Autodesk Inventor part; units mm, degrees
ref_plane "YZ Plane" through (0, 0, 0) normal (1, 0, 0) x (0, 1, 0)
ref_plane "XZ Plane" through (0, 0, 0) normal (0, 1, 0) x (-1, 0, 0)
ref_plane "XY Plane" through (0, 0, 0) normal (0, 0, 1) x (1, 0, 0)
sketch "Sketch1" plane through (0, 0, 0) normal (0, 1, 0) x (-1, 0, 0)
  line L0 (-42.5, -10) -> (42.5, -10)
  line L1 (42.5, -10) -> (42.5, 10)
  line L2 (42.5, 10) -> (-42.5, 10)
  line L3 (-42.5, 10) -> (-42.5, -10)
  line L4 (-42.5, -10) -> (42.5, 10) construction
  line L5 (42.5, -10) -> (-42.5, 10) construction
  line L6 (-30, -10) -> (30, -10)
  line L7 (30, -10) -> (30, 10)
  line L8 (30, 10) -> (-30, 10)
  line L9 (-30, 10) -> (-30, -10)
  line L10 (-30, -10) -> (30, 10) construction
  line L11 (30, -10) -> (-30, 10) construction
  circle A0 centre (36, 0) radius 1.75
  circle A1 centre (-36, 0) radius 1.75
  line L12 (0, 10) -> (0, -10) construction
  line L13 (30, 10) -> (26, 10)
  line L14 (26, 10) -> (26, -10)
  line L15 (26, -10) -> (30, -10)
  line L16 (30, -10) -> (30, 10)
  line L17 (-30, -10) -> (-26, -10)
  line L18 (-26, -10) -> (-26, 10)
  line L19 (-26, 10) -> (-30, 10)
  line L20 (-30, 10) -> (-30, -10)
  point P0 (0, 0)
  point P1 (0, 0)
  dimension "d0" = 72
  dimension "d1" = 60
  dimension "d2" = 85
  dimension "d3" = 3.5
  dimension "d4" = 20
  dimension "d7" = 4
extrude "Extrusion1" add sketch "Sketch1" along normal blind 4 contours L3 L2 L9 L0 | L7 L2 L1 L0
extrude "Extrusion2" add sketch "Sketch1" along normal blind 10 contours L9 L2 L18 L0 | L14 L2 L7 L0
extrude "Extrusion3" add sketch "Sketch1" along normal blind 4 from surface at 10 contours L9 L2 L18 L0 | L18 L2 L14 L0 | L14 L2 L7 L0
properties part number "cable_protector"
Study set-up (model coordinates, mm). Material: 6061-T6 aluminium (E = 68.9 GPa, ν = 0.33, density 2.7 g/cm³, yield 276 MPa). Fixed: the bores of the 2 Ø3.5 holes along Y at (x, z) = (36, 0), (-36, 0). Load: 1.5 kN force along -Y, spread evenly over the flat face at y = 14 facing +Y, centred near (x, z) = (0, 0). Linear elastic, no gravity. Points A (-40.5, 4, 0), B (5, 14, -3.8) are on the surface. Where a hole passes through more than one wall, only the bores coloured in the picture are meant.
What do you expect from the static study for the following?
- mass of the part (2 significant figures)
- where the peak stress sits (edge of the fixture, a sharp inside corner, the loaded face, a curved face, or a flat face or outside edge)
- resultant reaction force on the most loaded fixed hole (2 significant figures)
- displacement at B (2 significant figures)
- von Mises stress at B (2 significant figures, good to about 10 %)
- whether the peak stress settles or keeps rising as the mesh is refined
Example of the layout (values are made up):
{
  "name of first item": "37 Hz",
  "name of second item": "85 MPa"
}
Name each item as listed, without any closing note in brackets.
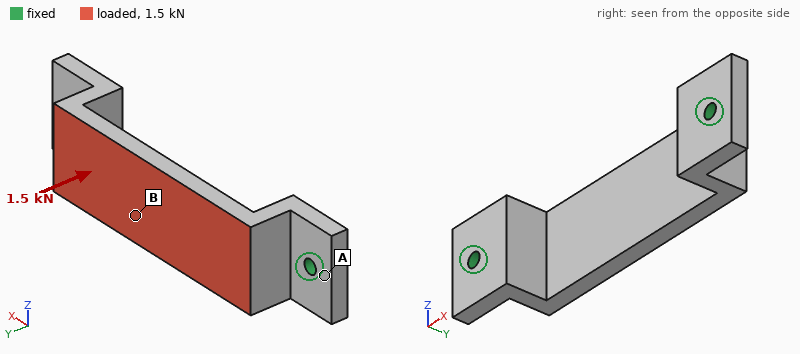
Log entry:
{
  "mass of the part": "22 g",
  "where the peak stress sits": "edge of the fixture",
  "resultant reaction force on the most loaded fixed hole": "1.2 kN",
  "displacement at B": "0.11 mm",
  "von Mises stress at B": "70 MPa",
  "whether the peak stress settles or keeps rising as the mesh is refined": "keeps rising"
}
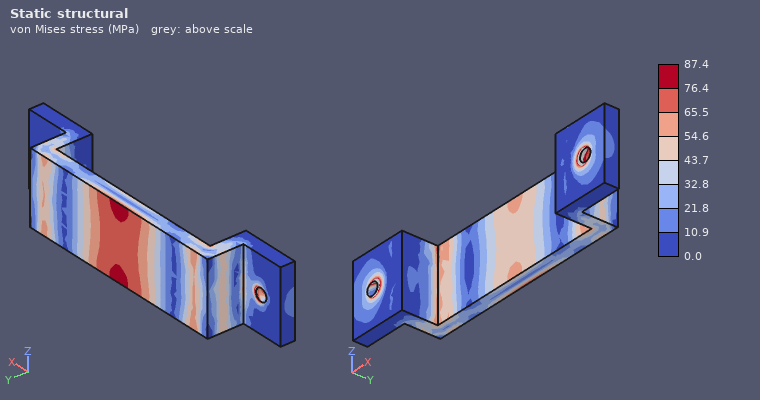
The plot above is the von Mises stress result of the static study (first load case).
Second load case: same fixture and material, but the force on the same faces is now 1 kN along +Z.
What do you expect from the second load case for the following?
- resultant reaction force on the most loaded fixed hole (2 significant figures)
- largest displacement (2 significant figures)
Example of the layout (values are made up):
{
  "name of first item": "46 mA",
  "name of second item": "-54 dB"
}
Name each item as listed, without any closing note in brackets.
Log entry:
{
  "resultant reaction force on the most loaded fixed hole": "500 N",
  "largest displacement": "91 µm"
}
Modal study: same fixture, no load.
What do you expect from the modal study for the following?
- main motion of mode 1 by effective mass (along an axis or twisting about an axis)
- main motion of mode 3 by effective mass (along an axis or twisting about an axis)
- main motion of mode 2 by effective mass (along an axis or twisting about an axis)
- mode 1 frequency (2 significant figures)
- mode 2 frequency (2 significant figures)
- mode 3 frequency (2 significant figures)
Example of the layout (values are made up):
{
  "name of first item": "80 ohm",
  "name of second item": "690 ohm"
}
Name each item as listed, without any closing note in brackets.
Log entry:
{
  "main motion of mode 1 by effective mass": "along Z",
  "main motion of mode 3 by effective mass": "along X",
  "main motion of mode 2 by effective mass": "along Y",
  "mode 1 frequency": "5300 Hz",
  "mode 2 frequency": "5700 Hz",
  "mode 3 frequency": "6600 Hz"
}
